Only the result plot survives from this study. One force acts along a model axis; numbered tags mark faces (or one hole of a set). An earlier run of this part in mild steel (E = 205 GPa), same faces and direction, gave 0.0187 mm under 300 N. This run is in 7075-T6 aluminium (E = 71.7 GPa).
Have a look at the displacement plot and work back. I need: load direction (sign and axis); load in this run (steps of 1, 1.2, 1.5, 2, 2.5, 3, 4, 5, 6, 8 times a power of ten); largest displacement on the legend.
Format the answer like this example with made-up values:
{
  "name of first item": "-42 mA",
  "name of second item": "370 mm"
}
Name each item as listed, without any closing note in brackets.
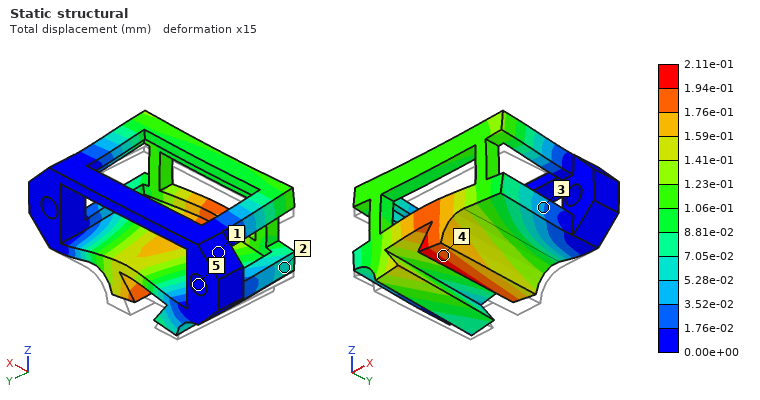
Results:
{
  "load direction": "+Z",
  "load in this run": "1.2 kN",
  "largest displacement on the legend": "2.11e-01 mm"
}
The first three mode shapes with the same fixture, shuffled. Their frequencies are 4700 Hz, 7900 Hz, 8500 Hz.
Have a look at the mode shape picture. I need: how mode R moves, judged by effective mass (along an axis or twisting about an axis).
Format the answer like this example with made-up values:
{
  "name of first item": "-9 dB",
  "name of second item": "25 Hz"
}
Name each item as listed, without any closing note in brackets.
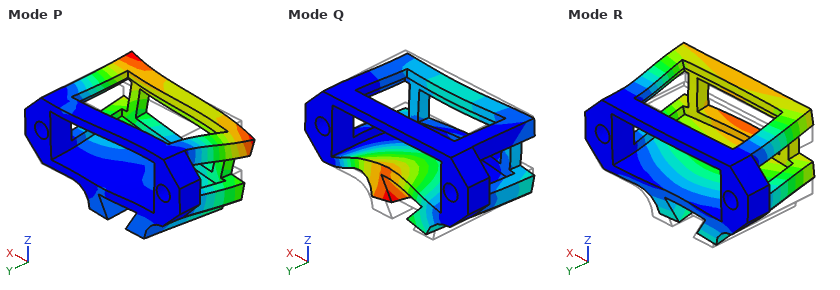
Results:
{
  "how mode R moves, judged by effective mass": "along Z"
}
